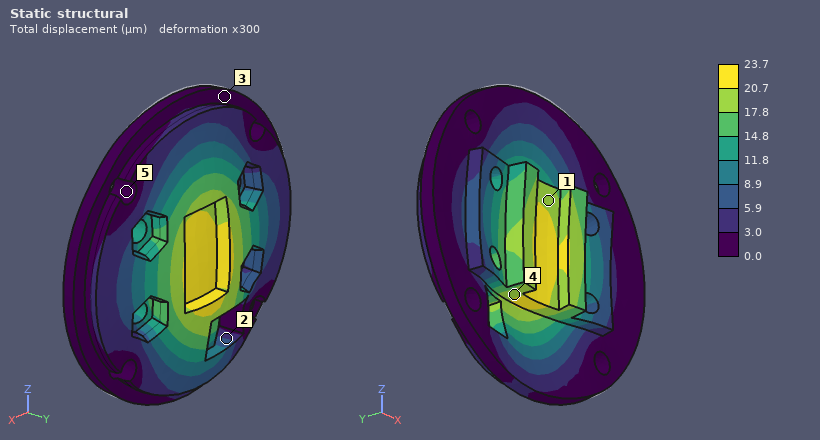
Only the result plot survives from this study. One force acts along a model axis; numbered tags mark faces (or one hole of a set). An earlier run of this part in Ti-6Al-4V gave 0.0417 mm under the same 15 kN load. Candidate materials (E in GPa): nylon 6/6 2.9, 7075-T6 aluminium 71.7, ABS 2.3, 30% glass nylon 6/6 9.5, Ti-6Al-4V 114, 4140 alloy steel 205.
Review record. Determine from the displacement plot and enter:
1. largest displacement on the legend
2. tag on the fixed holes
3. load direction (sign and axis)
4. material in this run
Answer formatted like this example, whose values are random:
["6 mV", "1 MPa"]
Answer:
["23.7 µm", "5", "+Y", "4140 alloy steel"]
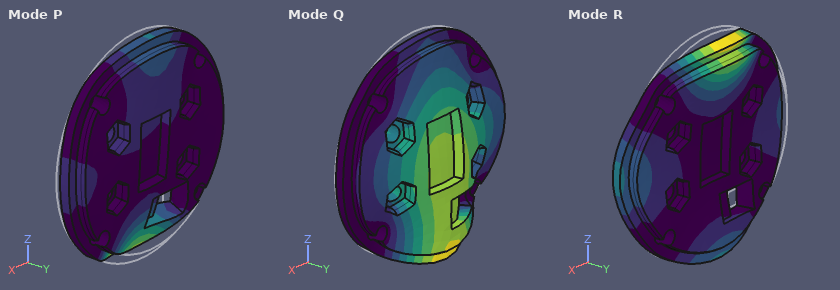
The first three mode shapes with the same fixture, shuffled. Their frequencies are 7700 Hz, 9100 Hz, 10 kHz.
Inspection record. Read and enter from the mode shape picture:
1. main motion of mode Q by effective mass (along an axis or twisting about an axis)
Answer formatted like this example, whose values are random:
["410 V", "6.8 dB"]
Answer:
["along Y"]
